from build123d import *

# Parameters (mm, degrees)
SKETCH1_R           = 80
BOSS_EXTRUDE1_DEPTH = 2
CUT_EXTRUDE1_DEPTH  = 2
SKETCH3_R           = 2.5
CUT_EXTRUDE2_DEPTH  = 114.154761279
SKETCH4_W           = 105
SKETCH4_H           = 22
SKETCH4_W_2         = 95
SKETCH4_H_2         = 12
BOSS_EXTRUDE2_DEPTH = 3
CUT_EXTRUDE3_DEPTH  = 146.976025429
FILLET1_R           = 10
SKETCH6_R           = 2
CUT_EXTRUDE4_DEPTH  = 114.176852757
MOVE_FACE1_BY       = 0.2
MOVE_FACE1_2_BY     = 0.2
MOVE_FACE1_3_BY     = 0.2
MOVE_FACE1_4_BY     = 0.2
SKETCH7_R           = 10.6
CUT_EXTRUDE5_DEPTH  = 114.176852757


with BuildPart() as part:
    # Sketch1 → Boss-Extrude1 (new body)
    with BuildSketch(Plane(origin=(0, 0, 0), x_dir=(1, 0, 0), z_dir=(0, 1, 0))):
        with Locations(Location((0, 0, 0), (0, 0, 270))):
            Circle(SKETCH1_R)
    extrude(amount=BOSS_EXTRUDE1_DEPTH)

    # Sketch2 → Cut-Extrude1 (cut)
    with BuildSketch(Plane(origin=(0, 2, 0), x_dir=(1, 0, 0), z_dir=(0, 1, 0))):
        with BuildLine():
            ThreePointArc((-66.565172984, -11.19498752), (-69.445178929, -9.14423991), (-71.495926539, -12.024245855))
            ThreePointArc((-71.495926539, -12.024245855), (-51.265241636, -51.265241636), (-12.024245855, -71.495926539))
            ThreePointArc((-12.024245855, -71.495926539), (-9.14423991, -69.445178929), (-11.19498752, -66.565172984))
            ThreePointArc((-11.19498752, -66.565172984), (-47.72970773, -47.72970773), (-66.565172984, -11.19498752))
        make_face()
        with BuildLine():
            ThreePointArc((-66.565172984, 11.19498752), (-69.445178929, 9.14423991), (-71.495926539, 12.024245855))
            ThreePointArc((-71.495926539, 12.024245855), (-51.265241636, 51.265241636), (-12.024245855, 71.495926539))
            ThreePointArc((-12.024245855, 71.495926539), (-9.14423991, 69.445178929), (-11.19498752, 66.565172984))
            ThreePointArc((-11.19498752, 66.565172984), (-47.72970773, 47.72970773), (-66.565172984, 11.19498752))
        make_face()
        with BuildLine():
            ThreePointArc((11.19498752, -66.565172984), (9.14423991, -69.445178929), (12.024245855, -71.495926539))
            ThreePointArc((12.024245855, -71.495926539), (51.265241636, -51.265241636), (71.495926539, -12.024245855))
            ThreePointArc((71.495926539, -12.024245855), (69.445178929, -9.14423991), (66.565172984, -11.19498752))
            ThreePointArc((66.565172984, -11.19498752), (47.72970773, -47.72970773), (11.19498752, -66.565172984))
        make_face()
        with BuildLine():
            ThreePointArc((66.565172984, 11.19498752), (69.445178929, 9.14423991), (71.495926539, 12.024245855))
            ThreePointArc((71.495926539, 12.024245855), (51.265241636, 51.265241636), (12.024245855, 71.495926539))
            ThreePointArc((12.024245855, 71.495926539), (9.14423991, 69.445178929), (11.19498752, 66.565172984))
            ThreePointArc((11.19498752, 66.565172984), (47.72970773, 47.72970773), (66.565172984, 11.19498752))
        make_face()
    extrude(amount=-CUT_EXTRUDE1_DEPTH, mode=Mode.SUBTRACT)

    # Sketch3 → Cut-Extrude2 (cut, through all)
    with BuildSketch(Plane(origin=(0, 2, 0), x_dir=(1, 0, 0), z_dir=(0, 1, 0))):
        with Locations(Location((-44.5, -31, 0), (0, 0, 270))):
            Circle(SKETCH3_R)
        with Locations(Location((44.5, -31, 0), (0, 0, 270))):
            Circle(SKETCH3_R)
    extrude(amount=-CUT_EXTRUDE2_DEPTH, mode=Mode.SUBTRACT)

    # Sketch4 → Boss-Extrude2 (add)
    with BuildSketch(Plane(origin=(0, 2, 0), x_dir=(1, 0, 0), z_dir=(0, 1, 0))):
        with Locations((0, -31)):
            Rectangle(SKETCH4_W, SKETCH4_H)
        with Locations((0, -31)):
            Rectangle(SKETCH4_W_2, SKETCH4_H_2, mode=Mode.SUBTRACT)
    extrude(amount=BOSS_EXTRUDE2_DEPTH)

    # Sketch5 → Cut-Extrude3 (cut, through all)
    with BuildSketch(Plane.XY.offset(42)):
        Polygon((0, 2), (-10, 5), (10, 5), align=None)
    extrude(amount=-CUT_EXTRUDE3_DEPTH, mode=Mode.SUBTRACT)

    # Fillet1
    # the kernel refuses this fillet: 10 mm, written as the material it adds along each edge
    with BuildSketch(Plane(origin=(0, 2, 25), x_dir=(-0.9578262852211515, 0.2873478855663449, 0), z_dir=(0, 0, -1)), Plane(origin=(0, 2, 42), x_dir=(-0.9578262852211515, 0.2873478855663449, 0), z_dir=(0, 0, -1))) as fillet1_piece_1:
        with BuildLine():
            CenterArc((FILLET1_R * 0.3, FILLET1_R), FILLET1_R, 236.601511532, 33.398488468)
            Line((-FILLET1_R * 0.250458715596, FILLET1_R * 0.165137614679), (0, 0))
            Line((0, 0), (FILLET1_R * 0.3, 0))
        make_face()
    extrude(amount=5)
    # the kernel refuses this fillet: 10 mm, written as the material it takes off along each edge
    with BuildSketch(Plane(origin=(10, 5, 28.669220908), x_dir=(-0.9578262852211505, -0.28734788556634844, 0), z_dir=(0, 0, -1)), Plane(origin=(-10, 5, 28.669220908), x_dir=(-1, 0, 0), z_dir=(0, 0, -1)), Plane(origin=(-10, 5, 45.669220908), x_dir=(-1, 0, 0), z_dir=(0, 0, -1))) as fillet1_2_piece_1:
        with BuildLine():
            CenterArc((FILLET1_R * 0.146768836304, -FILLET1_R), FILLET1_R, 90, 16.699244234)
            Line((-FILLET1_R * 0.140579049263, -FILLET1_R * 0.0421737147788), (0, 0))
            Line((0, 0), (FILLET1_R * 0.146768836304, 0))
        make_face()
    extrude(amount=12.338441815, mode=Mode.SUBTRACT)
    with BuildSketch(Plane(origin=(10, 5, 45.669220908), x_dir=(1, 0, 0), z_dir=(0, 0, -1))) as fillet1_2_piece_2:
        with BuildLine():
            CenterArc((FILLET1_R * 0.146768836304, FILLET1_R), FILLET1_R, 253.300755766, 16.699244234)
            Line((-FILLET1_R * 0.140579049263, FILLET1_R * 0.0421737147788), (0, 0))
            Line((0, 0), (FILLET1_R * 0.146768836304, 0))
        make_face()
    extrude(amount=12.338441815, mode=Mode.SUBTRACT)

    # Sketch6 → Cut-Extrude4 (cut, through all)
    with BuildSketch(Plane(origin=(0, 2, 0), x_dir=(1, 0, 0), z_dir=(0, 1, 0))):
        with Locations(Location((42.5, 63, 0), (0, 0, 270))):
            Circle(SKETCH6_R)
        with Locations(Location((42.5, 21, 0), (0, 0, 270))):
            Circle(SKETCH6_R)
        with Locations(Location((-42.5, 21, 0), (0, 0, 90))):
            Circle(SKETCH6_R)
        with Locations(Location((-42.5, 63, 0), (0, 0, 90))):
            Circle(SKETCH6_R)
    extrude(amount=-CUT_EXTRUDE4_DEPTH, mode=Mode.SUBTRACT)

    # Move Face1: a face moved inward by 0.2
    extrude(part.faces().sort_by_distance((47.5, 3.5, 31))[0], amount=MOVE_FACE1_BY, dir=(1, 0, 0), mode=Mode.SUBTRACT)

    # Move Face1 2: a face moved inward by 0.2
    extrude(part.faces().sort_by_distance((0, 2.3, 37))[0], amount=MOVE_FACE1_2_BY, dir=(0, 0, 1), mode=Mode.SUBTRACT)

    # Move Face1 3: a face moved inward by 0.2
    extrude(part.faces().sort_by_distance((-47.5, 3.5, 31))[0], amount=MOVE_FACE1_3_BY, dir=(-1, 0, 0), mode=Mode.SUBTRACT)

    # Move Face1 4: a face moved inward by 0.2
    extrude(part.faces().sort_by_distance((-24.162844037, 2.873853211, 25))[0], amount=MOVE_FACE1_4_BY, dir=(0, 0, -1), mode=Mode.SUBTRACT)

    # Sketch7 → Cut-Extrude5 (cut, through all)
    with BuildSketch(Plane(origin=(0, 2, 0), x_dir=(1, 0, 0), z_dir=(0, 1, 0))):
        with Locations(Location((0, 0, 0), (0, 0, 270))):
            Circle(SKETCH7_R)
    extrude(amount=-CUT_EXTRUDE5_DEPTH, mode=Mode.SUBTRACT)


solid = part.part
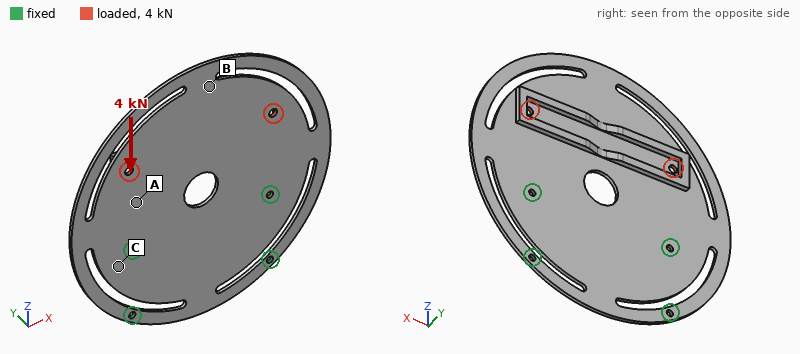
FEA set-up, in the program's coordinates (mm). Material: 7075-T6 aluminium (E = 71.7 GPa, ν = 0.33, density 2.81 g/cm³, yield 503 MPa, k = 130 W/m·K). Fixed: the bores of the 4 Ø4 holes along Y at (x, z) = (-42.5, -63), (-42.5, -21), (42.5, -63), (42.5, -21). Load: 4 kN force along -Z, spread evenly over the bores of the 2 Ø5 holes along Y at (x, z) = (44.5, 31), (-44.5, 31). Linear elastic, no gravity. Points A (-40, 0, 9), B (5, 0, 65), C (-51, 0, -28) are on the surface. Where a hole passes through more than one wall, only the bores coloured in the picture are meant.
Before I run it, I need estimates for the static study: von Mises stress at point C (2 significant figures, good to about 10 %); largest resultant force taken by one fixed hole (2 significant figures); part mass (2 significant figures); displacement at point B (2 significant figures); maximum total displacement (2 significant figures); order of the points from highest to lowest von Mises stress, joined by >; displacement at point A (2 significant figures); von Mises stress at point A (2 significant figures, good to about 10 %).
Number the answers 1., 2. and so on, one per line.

1. 13 MPa
2. 1.9 kN
3. 110 g
4. 31 µm
5. 39 µm
6. A > C > B
7. 15 µm
8. 27 MPa
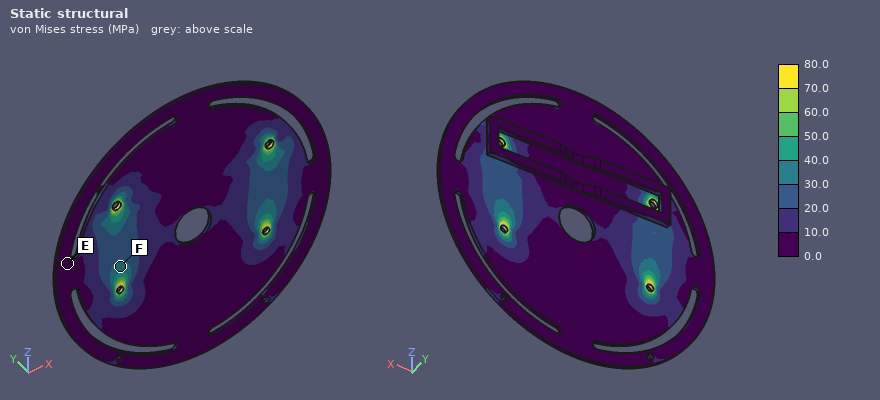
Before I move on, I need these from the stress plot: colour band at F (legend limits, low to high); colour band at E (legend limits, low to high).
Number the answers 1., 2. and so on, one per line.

1. 30.0 to 40.0 MPa
2. 0.0 to 10.0 MPa
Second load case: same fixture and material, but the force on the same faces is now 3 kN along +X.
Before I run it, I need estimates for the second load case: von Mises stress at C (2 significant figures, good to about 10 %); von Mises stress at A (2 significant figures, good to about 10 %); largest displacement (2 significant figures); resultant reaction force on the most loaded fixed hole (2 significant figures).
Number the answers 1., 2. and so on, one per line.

1. 23 MPa
2. 25 MPa
3. 69 µm
4. 2.2 kN
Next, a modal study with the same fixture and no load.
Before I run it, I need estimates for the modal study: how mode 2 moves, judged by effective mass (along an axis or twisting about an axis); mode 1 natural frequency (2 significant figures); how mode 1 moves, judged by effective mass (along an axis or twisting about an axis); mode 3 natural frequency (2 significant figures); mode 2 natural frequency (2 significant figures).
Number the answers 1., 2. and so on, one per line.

1. twisting about Z
2. 180 Hz
3. along Y
4. 740 Hz
5. 430 Hz
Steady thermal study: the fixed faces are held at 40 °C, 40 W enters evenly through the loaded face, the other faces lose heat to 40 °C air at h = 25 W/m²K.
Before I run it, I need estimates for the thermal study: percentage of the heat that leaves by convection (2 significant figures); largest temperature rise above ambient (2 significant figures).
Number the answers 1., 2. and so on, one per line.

1. 54 %
2. 64 K
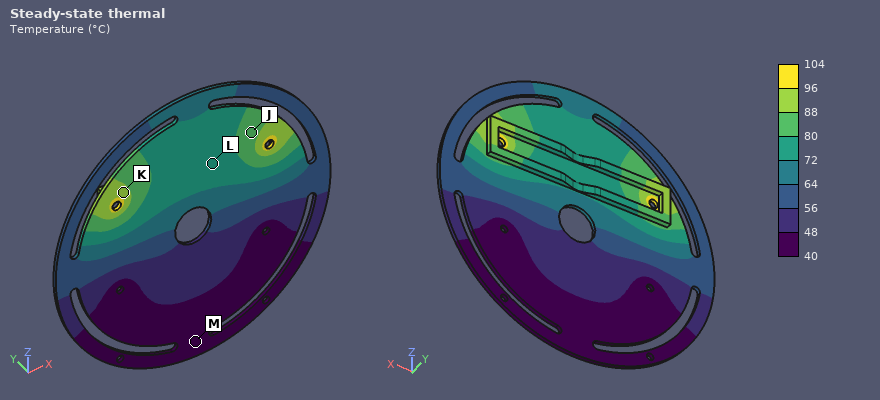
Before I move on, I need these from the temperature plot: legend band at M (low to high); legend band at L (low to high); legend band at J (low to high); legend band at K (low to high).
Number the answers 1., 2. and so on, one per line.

1. 40 to 48 °C
2. 72 to 80 °C
3. 80 to 88 °C
4. 88 to 96 °C
